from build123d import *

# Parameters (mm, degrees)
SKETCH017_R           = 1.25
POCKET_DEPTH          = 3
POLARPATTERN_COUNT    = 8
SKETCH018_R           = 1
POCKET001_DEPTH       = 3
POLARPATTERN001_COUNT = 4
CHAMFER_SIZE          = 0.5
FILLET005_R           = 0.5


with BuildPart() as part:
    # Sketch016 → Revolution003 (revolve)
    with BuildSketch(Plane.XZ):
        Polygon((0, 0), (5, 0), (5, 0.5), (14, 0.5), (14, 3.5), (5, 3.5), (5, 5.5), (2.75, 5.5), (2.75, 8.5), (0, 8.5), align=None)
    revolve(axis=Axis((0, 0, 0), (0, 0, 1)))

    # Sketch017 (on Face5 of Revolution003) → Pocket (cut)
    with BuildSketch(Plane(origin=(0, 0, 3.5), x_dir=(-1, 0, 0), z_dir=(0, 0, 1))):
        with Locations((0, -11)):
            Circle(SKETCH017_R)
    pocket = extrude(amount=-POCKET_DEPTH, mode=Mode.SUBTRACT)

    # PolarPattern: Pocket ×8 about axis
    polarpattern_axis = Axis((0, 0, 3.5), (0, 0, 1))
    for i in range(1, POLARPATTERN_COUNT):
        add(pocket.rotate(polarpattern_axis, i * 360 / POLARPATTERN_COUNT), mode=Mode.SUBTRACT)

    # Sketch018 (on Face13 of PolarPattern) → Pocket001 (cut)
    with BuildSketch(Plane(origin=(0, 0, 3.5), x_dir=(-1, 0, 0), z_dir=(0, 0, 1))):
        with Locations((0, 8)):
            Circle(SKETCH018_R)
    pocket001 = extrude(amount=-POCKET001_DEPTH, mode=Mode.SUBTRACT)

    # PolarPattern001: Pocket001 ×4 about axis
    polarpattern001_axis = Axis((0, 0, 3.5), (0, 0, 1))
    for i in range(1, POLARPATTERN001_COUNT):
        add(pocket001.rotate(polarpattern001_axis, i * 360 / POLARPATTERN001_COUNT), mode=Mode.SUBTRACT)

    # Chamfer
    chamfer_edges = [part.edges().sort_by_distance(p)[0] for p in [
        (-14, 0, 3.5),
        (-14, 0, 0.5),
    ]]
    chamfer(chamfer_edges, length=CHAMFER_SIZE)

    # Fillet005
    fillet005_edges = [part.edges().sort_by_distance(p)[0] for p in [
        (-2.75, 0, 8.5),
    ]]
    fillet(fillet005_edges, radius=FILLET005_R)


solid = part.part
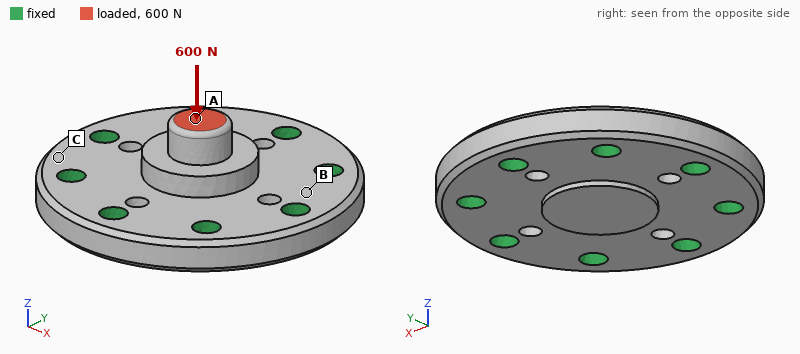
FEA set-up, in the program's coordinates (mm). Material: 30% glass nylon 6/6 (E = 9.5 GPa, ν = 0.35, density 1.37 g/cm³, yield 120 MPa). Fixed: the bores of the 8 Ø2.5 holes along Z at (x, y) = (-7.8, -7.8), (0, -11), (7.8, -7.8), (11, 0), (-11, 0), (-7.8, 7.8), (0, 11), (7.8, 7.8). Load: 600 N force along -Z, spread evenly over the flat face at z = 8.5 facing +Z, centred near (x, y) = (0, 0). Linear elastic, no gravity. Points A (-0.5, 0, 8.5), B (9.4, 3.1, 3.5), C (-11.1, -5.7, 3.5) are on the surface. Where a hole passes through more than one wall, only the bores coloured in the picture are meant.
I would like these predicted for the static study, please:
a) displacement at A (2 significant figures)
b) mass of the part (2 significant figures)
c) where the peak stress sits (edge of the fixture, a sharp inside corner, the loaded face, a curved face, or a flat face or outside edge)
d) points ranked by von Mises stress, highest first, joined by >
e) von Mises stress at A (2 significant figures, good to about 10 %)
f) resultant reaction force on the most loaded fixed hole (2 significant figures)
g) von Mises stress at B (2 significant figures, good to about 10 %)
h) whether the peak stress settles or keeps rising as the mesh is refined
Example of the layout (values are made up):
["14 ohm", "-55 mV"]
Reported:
["41 µm", "2.7 g", "edge of the fixture", "A > B > C", "23 MPa", "89 N", "9.3 MPa", "keeps rising"]
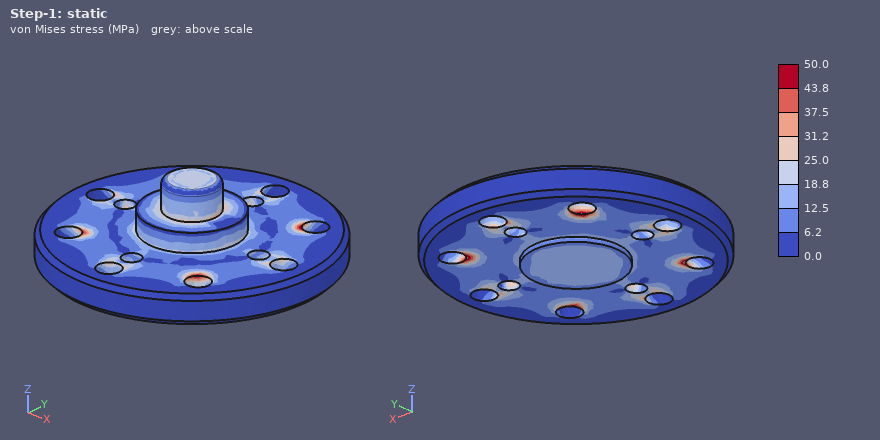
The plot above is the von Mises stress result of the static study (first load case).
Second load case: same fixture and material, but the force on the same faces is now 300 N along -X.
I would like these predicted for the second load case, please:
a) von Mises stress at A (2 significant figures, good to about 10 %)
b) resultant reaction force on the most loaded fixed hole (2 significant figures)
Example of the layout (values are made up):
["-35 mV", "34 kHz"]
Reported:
["33 MPa", "77 N"]
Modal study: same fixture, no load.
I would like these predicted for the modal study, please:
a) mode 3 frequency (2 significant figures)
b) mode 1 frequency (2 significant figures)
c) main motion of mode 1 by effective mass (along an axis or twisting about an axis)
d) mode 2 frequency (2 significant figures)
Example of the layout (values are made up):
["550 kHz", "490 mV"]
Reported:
["38 kHz", "25 kHz", "along Z", "38 kHz"]
